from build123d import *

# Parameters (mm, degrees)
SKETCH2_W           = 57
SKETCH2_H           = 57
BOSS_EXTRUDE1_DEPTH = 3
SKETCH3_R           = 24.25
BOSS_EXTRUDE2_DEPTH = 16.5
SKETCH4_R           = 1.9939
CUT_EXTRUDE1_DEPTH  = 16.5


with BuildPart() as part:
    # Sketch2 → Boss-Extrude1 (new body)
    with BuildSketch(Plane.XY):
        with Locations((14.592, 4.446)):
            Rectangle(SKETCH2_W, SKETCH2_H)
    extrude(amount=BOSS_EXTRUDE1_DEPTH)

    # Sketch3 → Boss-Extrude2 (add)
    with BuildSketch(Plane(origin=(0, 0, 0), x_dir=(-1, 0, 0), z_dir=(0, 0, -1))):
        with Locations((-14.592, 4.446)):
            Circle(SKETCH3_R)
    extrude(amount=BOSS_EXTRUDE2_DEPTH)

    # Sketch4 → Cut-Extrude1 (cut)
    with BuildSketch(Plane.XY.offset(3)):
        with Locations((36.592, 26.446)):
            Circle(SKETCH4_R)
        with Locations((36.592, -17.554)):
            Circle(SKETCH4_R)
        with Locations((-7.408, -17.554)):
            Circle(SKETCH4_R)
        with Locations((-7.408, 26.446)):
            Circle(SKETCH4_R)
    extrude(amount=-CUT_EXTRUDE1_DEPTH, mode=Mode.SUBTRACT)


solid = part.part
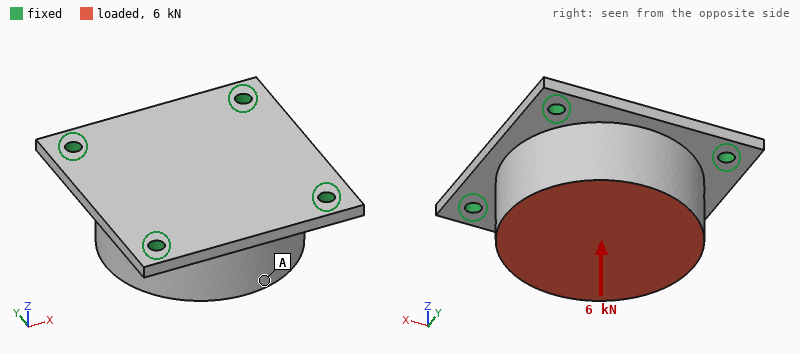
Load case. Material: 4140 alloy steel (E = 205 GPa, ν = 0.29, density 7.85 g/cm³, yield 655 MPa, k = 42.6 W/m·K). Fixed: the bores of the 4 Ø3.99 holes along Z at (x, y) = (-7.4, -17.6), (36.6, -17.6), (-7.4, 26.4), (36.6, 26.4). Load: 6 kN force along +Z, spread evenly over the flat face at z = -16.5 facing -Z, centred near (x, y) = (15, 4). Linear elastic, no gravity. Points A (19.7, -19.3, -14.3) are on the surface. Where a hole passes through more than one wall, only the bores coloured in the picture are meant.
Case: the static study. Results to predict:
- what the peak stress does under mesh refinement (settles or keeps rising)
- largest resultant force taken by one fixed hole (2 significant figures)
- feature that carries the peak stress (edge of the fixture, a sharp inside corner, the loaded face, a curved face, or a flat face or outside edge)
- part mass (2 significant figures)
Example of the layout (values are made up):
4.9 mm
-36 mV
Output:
keeps rising
1.7 kN
edge of the fixture
310 g
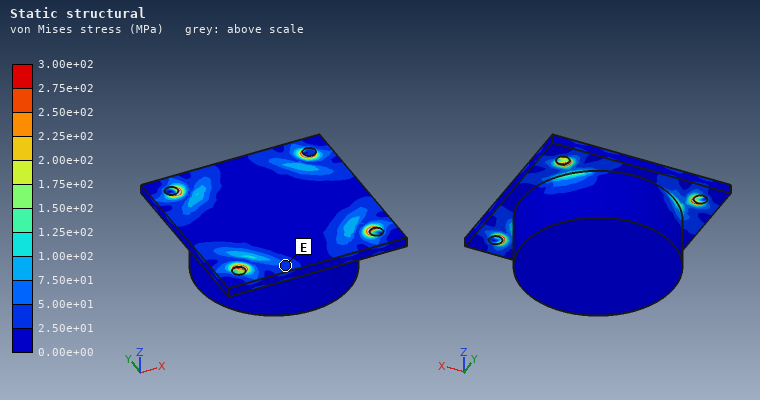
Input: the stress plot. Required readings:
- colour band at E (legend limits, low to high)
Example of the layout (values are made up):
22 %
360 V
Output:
2.50e+01 to 5.00e+01 MPa
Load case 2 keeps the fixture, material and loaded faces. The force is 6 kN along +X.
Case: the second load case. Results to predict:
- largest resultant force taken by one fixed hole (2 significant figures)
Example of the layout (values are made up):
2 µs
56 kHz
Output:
2.2 kN
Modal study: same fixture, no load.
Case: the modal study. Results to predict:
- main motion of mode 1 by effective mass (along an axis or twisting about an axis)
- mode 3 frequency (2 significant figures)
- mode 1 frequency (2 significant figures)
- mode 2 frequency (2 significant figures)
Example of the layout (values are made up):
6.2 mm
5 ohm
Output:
along Z
7600 Hz
6200 Hz
7500 Hz
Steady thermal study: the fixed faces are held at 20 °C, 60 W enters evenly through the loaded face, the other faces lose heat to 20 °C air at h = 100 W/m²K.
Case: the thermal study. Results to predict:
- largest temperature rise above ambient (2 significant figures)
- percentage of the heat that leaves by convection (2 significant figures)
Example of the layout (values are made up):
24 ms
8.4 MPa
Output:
52 K
41 %
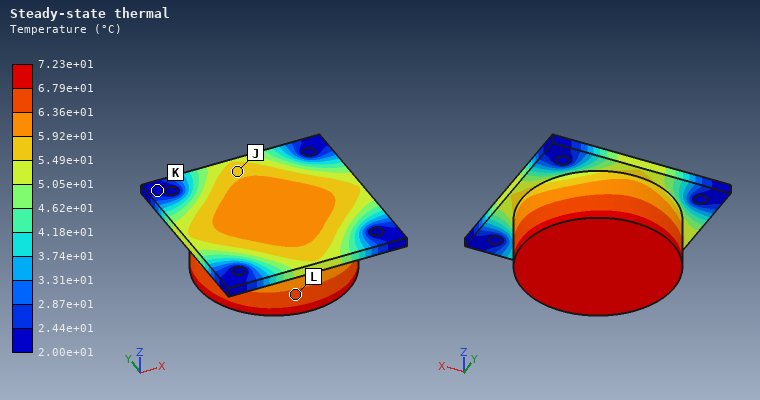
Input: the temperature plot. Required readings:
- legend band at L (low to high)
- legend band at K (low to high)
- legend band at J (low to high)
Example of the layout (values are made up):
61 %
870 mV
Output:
6.36e+01 to 6.79e+01 °C
2.00e+01 to 2.44e+01 °C
5.49e+01 to 5.92e+01 °C
